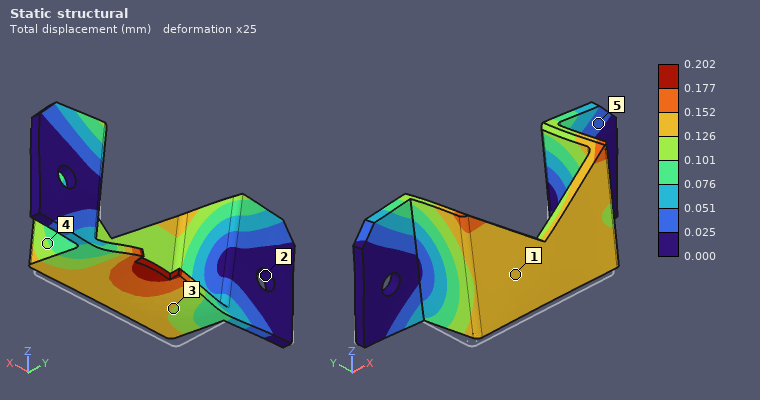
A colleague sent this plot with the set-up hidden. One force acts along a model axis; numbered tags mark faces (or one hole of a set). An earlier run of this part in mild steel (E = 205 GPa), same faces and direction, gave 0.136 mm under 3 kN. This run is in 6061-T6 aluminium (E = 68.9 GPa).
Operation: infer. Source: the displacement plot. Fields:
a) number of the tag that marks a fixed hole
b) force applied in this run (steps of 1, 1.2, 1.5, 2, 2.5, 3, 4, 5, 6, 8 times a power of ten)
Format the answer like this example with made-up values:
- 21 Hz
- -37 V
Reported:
- 2
- 1.5 kN
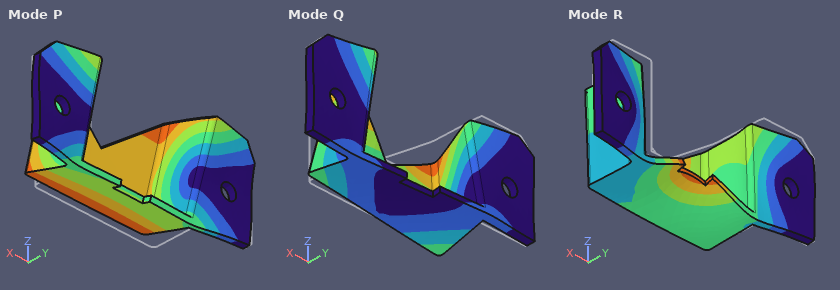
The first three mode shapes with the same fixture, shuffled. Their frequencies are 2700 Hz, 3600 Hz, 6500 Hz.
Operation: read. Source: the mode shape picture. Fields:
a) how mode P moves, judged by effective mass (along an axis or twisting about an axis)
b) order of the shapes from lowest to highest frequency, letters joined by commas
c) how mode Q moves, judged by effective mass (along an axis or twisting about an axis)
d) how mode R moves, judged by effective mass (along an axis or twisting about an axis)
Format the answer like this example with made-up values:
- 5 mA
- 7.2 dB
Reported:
- along Z
- P, Q, R
- along X
- along Y
